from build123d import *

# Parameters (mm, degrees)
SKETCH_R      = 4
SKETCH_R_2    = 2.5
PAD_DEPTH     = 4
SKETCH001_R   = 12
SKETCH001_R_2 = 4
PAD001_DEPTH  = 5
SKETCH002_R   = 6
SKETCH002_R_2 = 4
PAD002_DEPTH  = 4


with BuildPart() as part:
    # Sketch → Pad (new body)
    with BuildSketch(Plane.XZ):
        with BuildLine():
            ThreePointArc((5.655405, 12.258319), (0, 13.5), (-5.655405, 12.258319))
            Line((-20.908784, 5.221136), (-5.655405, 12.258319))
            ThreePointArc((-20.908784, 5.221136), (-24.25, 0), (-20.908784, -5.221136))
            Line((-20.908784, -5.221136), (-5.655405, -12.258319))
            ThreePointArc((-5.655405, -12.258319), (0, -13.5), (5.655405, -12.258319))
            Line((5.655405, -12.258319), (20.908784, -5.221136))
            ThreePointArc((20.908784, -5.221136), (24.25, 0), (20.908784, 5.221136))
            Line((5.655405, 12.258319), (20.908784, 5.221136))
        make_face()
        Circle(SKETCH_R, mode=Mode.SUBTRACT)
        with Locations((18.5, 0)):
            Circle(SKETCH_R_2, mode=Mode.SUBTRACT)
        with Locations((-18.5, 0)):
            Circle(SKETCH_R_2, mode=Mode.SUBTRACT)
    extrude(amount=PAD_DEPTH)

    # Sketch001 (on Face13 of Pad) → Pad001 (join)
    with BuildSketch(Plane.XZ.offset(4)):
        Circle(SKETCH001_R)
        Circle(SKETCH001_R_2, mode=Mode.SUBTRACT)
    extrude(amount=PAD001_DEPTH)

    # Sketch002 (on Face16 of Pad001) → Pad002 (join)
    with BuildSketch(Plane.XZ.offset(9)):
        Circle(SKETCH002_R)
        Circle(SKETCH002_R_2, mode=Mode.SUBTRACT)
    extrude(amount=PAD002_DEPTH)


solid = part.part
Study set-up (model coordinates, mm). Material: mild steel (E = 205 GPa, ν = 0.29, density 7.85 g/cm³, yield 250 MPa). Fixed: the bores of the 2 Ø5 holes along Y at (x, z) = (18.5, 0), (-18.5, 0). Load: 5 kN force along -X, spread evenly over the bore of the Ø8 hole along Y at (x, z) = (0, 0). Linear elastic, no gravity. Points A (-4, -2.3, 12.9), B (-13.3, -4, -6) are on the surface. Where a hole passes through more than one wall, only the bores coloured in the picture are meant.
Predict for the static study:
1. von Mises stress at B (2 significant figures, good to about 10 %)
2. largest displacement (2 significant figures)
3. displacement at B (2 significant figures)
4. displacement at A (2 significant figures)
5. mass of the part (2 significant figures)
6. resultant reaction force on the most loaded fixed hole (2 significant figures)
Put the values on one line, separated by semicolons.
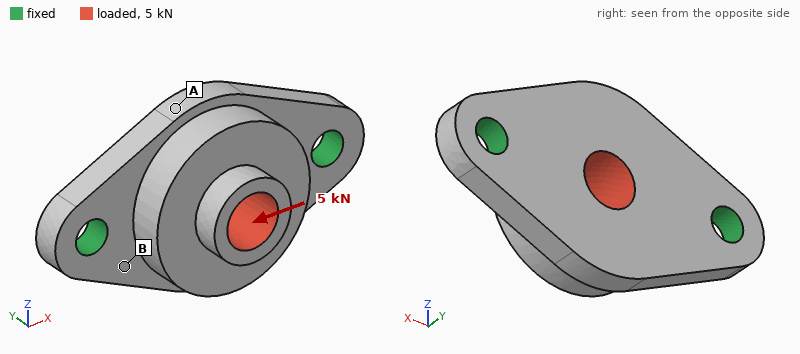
45 MPa; 7.3 µm; 2.0 µm; 2.1 µm; 43 g; 2.6 kN
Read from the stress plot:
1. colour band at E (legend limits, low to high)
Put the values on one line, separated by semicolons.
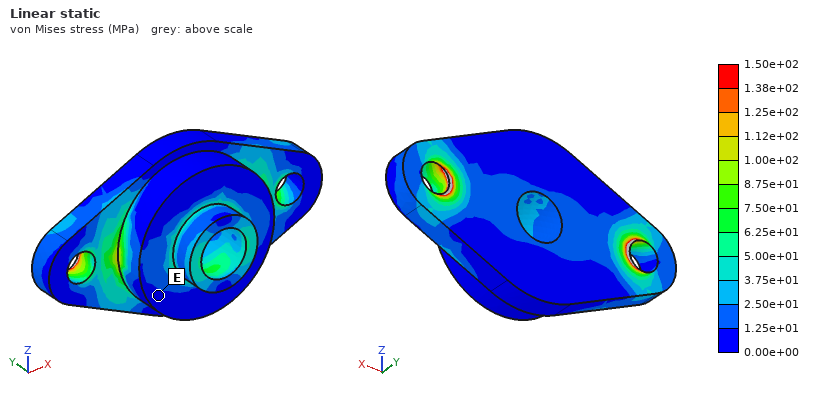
0.00e+00 to 1.25e+01 MPa
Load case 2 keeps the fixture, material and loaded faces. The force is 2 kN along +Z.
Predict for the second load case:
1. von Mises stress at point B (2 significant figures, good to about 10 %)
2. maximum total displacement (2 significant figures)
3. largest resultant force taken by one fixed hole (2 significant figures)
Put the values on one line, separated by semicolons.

60 MPa; 17 µm; 1.0 kN
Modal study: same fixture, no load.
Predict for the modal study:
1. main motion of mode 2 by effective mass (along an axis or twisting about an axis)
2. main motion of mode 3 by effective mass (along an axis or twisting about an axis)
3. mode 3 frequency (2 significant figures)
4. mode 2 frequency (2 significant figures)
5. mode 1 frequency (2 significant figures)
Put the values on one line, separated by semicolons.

along Y; along Z; 26 kHz; 15 kHz; 9800 Hz
